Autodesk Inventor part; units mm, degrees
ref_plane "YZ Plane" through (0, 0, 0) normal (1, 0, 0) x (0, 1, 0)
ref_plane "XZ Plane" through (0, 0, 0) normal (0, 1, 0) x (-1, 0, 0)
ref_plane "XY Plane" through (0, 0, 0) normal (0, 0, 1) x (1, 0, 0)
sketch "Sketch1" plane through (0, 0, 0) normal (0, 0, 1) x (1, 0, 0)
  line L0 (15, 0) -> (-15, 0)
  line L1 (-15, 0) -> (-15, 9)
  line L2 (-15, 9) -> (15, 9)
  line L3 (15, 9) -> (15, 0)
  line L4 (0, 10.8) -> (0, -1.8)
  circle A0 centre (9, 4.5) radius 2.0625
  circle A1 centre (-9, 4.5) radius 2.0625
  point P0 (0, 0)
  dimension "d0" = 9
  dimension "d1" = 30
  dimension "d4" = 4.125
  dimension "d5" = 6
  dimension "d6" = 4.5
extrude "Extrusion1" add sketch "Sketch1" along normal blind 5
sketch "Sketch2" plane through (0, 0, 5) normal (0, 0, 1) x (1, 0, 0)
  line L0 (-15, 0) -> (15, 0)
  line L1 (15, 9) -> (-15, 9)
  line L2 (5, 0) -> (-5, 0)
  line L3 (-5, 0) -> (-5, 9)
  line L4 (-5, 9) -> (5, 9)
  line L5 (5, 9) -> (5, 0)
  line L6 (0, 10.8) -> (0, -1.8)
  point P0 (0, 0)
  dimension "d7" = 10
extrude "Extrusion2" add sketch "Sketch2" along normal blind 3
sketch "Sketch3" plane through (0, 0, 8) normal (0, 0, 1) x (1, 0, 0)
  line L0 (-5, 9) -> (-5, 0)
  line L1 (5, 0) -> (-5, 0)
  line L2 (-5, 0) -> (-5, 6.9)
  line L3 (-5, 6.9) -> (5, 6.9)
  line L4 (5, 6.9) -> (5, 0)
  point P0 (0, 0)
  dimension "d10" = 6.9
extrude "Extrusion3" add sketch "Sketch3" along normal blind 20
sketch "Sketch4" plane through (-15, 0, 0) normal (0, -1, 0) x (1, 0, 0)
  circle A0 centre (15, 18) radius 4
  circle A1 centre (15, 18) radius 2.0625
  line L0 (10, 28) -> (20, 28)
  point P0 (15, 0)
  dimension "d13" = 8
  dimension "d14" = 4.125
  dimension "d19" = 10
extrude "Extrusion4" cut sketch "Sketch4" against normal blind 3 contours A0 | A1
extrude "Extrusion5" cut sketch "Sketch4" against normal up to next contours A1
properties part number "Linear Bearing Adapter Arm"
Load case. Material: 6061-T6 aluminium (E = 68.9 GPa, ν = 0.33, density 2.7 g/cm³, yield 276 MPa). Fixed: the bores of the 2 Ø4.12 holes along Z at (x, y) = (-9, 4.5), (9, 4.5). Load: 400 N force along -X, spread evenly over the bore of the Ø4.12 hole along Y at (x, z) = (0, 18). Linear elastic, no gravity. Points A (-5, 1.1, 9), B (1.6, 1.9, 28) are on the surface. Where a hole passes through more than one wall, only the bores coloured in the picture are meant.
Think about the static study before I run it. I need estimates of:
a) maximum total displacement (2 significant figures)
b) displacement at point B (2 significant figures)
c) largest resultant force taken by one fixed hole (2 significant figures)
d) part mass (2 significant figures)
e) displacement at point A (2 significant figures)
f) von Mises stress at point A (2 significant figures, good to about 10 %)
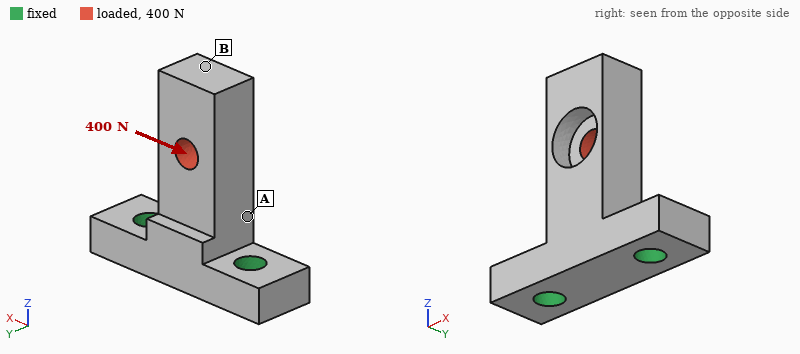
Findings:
35 µm
33 µm
500 N
7.2 g
6.2 µm
28 MPa
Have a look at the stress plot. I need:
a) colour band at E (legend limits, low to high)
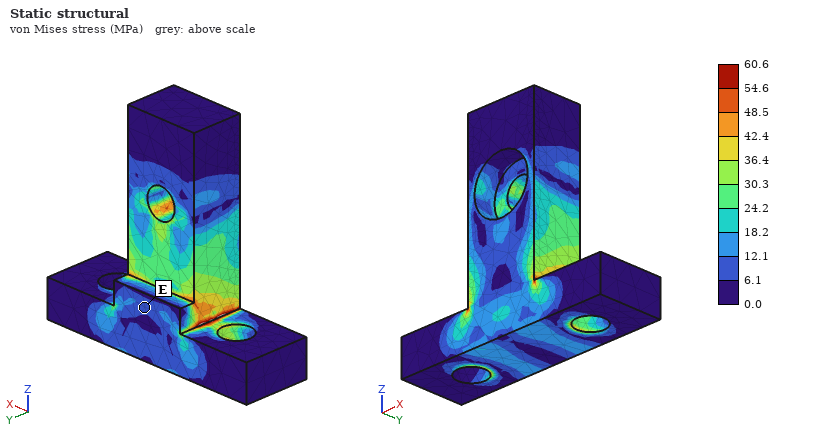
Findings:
6.1 to 12.1 MPa
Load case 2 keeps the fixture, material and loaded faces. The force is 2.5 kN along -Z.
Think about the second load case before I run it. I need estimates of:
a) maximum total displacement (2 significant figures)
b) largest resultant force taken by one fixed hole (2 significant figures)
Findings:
52 µm
1.3 kN
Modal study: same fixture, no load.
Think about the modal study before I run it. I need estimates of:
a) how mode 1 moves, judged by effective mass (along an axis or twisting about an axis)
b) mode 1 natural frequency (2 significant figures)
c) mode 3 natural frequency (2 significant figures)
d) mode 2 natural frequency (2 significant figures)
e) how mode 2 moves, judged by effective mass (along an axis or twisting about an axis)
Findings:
along Y
6900 Hz
25 kHz
11 kHz
along X
